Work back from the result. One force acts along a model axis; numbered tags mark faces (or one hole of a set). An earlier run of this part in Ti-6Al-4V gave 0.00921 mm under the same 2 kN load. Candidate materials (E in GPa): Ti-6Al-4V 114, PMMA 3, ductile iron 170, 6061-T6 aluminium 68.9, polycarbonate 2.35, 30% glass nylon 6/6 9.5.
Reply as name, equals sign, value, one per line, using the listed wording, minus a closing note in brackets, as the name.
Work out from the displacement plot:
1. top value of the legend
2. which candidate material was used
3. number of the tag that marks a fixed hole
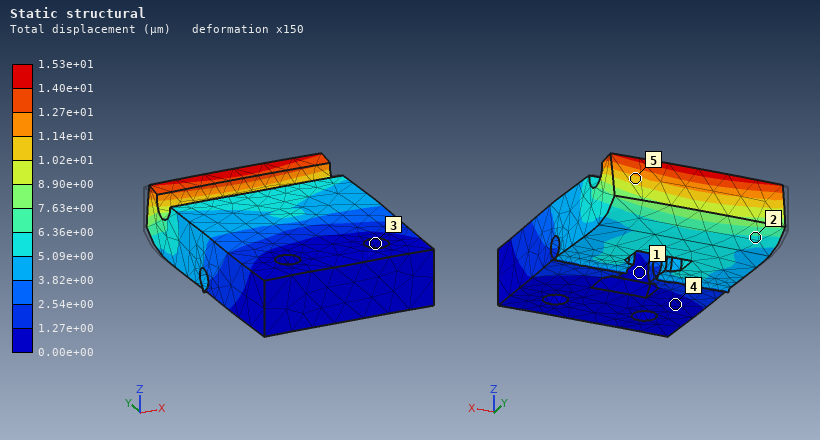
top value of the legend = 1.53e+01 µm
which candidate material was used = 6061-T6 aluminium
number of the tag that marks a fixed hole = 3
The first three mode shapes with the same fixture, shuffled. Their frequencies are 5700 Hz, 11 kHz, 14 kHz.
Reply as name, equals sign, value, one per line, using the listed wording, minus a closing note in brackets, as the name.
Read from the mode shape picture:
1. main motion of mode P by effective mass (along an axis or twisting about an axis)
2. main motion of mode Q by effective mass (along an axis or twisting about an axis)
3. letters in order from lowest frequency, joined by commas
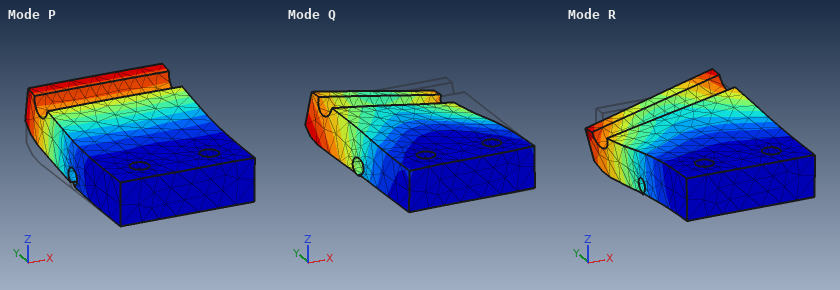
main motion of mode P by effective mass = along Z
main motion of mode Q by effective mass = along X
letters in order from lowest frequency, joined by commas = P, Q, R
